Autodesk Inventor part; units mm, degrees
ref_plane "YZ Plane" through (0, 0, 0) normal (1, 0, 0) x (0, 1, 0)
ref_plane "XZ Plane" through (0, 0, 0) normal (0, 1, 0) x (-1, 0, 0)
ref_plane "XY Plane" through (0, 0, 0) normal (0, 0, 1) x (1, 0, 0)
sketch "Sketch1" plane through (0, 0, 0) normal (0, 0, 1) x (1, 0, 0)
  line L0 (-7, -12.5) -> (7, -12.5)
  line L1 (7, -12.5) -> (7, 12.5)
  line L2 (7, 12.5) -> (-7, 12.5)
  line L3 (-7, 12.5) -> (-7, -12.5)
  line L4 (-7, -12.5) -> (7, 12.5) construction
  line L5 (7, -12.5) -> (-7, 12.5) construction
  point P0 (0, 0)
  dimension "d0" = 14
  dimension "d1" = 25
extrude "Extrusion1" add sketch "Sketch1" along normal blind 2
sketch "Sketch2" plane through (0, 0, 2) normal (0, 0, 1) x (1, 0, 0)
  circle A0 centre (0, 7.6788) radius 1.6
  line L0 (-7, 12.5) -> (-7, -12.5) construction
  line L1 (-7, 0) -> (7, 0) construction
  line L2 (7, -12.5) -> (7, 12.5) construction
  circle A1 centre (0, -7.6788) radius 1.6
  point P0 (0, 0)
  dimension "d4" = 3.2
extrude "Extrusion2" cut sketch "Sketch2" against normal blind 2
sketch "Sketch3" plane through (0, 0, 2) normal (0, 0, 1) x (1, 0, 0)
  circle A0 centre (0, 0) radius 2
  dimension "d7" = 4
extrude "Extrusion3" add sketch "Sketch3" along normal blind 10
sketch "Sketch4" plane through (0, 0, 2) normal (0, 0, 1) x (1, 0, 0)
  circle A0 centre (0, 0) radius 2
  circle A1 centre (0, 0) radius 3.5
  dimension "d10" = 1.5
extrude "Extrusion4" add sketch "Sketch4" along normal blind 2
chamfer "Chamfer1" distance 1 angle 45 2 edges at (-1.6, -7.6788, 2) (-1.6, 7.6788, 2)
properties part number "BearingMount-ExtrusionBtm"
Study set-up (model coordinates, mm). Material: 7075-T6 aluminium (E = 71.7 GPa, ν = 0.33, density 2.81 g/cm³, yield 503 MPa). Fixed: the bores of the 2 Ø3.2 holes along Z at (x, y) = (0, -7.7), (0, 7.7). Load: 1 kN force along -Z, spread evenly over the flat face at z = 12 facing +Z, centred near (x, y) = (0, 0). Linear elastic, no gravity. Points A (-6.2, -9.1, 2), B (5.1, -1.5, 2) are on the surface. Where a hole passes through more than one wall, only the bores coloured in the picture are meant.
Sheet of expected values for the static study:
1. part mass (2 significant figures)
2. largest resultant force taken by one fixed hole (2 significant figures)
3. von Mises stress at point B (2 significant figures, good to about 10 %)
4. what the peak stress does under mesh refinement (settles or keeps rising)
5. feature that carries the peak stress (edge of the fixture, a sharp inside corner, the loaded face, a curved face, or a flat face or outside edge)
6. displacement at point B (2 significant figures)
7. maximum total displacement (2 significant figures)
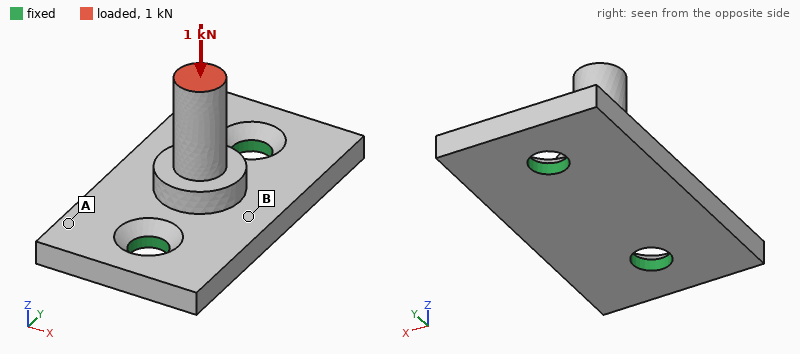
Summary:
2.3 g
660 N
59 MPa
keeps rising
edge of the fixture
22 µm
31 µm
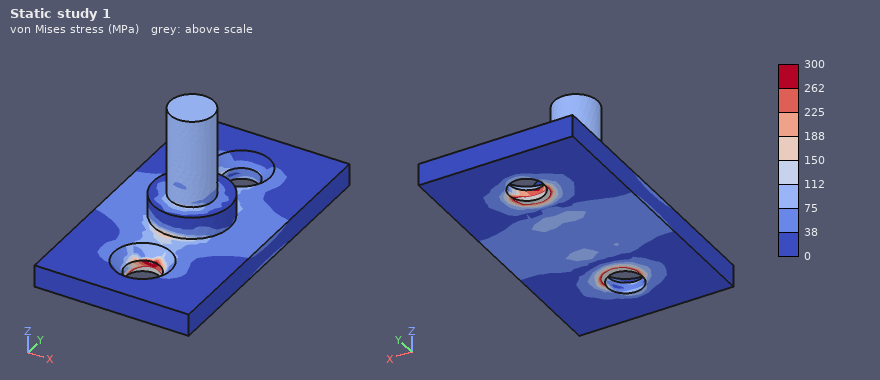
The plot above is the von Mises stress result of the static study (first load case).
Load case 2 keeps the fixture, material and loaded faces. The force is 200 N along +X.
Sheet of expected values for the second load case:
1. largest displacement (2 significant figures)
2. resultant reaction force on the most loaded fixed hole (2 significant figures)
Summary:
0.14 mm
100 N
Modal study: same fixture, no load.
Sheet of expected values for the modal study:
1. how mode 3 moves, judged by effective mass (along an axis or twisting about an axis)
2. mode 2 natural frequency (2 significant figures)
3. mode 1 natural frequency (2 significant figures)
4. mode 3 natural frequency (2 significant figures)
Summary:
along Z
27 kHz
15 kHz
29 kHz
